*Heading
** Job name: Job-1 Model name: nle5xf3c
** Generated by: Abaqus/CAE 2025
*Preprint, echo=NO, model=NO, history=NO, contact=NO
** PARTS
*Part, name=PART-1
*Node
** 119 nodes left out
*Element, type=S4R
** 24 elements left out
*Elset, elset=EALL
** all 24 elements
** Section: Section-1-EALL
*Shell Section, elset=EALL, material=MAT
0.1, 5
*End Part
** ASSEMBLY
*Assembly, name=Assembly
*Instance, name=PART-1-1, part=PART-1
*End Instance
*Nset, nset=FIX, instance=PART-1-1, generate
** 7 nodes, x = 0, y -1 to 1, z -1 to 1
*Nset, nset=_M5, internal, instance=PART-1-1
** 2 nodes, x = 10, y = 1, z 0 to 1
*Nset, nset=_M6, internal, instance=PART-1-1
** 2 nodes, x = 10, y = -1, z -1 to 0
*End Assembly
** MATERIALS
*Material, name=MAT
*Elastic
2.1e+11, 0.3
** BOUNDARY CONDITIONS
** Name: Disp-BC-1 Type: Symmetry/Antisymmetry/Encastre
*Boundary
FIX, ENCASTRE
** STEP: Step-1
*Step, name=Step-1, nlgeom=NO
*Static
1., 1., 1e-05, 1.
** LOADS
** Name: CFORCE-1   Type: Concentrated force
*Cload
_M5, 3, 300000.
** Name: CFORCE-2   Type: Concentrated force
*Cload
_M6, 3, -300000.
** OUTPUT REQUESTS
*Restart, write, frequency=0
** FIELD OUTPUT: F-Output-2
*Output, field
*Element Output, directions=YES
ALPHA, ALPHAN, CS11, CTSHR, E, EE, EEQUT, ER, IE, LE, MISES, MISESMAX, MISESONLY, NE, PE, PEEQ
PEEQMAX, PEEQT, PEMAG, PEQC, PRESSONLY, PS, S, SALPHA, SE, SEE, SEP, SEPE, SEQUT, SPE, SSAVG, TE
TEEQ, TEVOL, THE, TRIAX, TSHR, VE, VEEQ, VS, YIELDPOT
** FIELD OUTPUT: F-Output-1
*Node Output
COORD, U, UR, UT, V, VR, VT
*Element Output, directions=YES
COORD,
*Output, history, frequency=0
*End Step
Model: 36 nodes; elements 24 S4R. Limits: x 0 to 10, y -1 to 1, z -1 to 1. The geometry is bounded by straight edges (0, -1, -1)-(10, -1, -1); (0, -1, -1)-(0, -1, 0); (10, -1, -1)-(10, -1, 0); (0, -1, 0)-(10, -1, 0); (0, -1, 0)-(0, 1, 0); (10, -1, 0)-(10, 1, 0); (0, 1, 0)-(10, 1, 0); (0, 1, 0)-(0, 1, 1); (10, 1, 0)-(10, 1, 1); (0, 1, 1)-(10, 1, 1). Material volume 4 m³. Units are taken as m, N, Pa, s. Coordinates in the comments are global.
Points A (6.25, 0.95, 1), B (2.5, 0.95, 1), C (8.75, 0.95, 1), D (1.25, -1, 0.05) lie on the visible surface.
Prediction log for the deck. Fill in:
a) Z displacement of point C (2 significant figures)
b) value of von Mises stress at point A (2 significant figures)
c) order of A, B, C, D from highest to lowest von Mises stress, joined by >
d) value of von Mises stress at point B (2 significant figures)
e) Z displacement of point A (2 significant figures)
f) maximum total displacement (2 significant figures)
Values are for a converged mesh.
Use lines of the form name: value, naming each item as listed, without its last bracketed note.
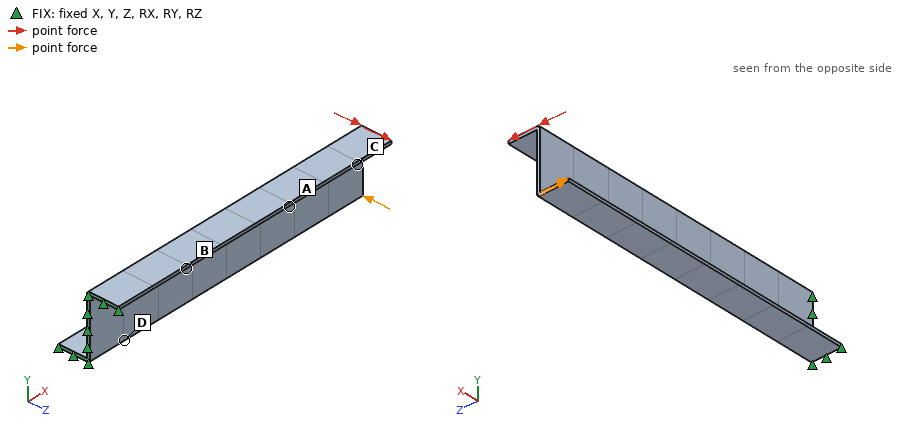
Z displacement of point C: 0.025 m
value of von Mises stress at point A: 7.3e+07 Pa
order of A, B, C, D from highest to lowest von Mises stress, joined by >: B > A > D > C
value of von Mises stress at point B: 1.2e+08 Pa
Z displacement of point A: 0.014 m
maximum total displacement: 0.044 m
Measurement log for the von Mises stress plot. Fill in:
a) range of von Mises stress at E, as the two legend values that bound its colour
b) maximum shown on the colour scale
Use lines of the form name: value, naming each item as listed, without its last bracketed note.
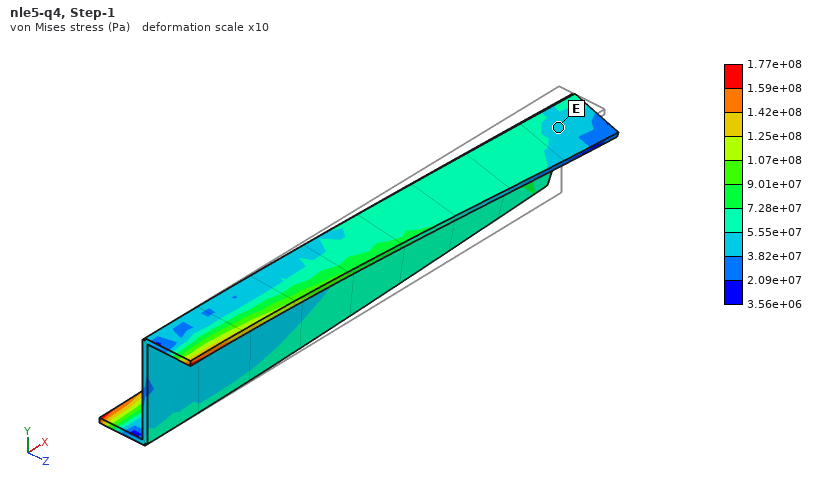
range of von Mises stress at E, as the two legend values that bound its colour: 3.82e+07 to 5.55e+07 Pa
maximum shown on the colour scale: 1.77e+08 Pa
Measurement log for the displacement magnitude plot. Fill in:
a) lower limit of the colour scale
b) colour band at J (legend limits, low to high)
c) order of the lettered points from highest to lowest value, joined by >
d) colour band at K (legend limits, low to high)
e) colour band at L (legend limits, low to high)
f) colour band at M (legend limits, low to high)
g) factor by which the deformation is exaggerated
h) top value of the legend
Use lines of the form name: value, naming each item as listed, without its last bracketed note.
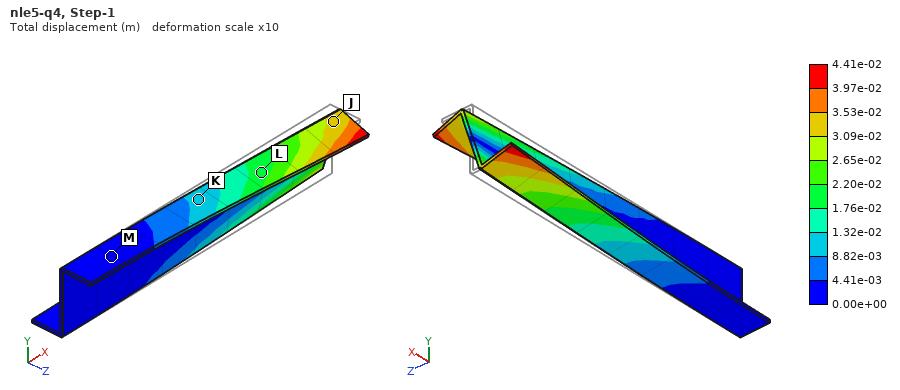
lower limit of the colour scale: 0.00e+00 m
colour band at J: 3.09e-02 to 3.53e-02 m
order of the lettered points from highest to lowest value, joined by >: J > L > K > M
colour band at K: 8.82e-03 to 1.32e-02 m
colour band at L: 1.76e-02 to 2.20e-02 m
colour band at M: 0.00e+00 to 4.41e-03 m
factor by which the deformation is exaggerated: 10
top value of the legend: 4.41e-02 m
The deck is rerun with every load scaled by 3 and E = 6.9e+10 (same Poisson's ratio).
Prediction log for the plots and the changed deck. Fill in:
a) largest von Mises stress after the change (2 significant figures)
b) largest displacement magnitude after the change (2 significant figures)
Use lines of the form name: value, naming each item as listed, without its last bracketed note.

largest von Mises stress after the change: 5.3e+08 Pa
largest displacement magnitude after the change: 0.40 m
